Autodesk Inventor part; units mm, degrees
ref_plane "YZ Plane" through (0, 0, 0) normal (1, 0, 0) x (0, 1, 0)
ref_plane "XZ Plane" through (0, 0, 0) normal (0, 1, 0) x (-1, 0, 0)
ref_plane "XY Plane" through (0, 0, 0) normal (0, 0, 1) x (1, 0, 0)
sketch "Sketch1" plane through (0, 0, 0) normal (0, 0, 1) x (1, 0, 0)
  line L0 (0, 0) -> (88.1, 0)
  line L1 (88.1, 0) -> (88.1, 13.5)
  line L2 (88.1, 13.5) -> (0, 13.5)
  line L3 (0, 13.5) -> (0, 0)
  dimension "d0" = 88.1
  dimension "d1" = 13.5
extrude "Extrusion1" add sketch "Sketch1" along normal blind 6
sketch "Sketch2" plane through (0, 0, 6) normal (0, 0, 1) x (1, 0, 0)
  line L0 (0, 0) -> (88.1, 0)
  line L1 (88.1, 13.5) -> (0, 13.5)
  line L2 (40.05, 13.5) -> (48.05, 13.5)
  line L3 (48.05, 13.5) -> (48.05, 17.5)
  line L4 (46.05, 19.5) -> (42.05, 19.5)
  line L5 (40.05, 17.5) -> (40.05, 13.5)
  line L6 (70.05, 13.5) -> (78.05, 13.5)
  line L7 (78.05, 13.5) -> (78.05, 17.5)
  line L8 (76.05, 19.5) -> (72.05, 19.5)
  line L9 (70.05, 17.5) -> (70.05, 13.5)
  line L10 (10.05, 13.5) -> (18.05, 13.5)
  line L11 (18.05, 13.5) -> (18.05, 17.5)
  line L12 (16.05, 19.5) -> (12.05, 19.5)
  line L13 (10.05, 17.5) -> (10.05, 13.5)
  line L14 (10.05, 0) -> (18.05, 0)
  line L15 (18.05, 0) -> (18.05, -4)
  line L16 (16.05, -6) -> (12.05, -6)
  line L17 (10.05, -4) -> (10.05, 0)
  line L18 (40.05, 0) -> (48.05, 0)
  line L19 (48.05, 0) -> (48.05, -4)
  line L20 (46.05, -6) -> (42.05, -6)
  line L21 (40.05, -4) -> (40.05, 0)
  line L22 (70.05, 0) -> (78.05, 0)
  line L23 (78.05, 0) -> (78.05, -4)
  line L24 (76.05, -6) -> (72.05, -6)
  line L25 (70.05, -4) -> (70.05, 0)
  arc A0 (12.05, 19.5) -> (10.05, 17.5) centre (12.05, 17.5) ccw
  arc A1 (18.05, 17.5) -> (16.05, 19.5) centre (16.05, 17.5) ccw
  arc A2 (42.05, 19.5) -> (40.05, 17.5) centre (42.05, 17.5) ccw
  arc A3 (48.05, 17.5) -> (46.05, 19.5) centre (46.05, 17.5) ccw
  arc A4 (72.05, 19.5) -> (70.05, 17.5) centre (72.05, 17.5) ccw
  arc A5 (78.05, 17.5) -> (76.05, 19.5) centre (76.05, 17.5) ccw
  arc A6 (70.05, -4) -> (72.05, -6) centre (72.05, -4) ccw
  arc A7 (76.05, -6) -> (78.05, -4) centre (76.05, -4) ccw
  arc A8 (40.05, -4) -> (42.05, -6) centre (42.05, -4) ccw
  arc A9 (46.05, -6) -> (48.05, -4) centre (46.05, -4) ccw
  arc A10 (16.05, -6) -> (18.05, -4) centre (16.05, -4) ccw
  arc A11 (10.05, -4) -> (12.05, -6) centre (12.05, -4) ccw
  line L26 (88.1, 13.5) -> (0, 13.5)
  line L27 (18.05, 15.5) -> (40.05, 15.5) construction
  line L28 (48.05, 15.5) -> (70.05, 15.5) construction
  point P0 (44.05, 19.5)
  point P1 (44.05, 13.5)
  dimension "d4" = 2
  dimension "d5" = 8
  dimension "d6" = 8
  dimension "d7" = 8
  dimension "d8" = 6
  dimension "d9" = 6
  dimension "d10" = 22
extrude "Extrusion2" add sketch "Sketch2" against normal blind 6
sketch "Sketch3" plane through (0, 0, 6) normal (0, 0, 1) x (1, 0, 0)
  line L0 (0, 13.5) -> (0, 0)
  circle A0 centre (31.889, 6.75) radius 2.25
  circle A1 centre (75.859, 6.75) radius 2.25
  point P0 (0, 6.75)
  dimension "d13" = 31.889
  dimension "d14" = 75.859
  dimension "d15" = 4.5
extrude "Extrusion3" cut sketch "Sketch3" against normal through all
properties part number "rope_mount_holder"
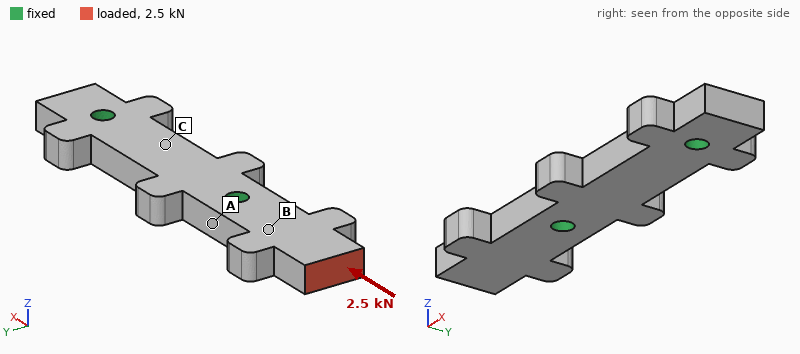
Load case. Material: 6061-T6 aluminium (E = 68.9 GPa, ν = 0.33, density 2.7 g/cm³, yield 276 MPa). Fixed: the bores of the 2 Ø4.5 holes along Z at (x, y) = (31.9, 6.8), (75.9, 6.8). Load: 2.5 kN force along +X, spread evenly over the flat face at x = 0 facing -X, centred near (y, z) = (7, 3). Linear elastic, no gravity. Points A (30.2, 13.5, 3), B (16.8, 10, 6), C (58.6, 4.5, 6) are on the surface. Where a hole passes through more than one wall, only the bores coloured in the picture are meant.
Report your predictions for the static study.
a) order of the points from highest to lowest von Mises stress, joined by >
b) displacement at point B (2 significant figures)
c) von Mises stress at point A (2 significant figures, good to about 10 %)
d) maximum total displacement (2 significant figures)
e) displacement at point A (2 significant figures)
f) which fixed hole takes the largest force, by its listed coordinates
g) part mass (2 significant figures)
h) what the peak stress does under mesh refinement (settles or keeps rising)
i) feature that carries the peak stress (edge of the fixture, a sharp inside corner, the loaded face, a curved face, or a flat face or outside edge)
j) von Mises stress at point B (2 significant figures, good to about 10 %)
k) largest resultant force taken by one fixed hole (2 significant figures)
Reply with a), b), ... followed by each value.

a) B > A > C
b) 6.9 µm
c) 16 MPa
d) 14 µm
e) 2.2 µm
f) (31.9, 6.8)
g) 23 g
h) keeps rising
i) edge of the fixture
j) 30 MPa
k) 2.4 kN
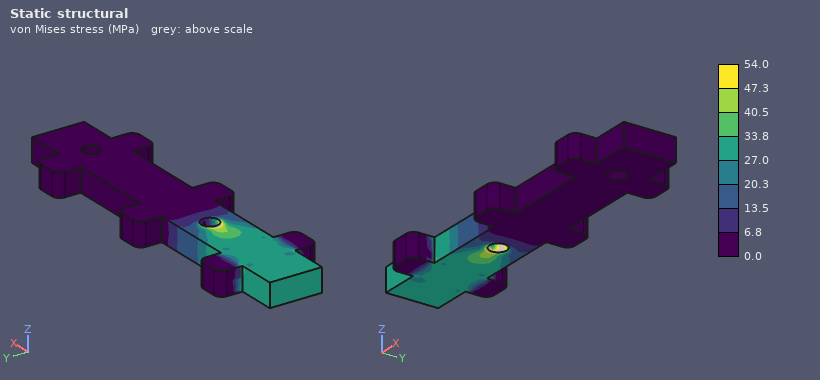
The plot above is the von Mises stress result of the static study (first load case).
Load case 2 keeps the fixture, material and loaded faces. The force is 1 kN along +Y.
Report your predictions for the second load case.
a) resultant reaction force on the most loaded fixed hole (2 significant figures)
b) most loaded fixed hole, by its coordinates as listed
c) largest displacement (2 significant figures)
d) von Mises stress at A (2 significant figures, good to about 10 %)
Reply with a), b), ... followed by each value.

a) 1.3 kN
b) (31.9, 6.8)
c) 0.20 mm
d) 140 MPa
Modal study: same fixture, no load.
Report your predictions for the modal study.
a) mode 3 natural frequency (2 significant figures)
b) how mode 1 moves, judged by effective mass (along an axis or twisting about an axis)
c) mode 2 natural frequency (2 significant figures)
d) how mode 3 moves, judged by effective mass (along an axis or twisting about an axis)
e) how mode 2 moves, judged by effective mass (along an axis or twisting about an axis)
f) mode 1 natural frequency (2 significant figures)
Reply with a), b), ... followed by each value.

a) 11 kHz
b) along Z
c) 7200 Hz
d) twisting about X
e) along Y
f) 4600 Hz
